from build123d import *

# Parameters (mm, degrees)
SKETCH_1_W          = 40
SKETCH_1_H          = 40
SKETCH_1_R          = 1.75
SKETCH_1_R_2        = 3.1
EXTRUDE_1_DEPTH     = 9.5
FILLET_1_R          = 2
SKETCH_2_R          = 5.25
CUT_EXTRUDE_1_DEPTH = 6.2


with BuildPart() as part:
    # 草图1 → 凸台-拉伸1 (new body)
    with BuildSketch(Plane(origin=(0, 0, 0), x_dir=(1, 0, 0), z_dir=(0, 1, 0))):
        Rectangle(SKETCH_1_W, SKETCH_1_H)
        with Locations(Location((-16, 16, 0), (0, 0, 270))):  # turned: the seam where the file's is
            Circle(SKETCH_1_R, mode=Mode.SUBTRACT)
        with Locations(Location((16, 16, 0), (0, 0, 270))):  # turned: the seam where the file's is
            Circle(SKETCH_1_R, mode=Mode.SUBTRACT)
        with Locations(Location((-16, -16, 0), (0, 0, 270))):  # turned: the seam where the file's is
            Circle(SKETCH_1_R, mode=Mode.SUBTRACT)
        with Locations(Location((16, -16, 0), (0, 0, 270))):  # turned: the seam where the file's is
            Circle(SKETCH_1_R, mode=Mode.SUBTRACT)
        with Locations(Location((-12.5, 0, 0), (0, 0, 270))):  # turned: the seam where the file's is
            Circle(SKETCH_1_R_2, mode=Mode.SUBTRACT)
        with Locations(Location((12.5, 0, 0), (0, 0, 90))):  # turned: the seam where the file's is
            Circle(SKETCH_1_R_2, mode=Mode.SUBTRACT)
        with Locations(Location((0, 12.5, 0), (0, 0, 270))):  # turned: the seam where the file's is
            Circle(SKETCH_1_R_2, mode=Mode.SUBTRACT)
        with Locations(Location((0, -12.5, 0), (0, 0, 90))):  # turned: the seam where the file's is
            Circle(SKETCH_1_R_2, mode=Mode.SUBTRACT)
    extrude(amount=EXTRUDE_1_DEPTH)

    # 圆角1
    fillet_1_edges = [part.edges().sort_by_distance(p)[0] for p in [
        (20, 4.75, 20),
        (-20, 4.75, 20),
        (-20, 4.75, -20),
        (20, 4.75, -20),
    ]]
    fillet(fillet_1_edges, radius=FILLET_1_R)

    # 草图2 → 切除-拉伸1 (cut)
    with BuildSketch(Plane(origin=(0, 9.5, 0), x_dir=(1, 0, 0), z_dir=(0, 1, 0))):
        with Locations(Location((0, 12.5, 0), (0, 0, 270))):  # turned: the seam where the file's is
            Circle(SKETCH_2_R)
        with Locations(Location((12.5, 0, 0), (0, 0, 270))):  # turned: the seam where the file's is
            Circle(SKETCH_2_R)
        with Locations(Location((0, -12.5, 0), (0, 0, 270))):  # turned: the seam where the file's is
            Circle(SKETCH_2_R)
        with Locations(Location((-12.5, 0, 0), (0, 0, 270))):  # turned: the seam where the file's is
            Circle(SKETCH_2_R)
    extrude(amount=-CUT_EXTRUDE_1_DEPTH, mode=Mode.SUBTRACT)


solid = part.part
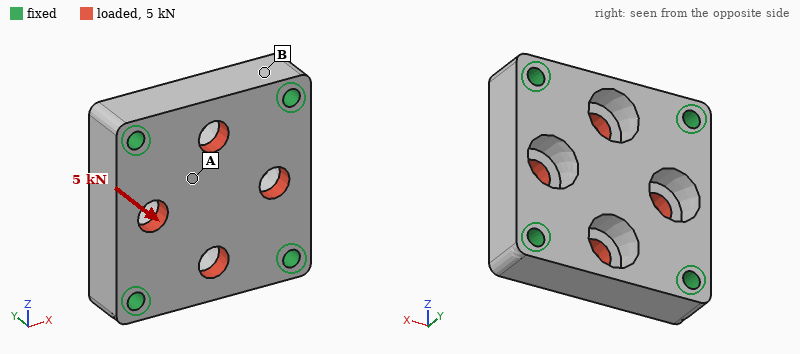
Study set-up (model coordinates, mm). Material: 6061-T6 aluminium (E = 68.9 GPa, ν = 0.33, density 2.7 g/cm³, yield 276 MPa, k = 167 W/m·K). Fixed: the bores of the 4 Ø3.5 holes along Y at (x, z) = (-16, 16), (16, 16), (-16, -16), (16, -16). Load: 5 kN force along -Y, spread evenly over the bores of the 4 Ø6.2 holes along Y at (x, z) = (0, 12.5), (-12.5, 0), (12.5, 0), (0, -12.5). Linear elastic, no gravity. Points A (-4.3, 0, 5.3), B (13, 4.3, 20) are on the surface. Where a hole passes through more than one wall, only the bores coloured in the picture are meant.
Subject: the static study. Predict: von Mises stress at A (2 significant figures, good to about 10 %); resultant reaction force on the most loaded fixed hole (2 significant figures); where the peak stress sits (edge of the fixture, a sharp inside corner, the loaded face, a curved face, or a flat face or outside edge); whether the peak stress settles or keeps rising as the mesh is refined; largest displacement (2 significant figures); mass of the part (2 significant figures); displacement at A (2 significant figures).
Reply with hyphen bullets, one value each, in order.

- 23 MPa
- 1.3 kN
- edge of the fixture
- keeps rising
- 16 µm
- 33 g
- 12 µm
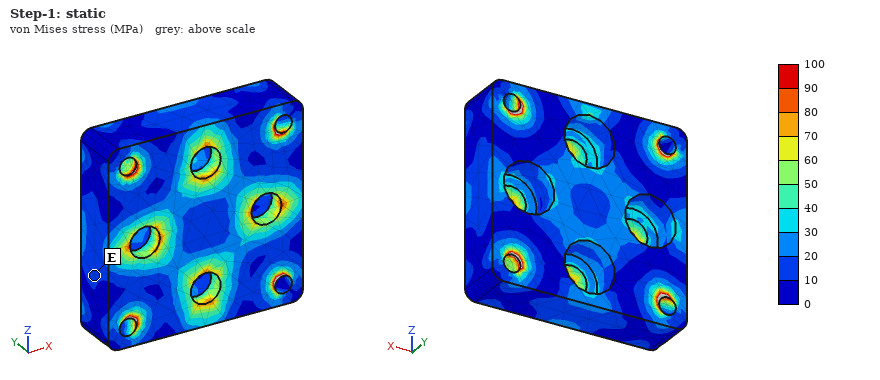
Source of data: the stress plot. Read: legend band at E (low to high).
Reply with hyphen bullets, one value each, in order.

- 10 to 20 MPa
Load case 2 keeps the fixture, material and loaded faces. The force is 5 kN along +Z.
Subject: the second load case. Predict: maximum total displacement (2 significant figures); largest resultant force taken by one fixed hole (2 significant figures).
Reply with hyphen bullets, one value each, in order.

- 8.0 µm
- 1.3 kN
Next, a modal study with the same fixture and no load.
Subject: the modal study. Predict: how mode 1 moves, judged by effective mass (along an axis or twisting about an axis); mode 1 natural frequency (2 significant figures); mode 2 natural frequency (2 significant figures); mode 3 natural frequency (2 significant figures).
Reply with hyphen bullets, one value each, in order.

- along Y
- 24 kHz
- 38 kHz
- 38 kHz
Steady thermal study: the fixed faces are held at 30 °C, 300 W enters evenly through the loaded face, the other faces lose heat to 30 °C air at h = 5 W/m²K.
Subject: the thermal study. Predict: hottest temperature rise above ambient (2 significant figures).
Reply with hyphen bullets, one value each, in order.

- 55 K
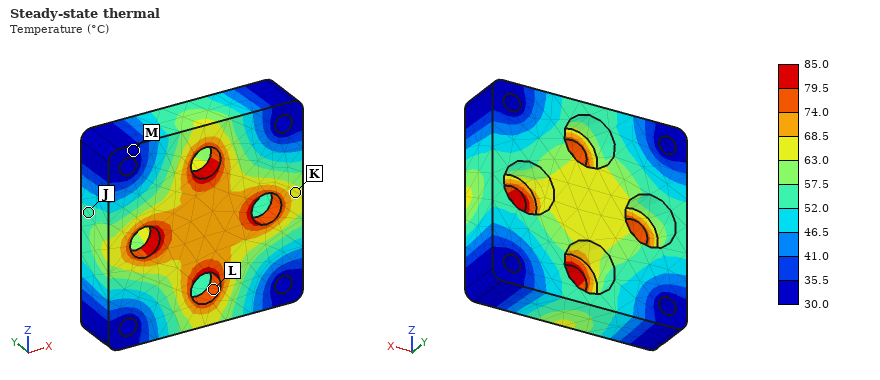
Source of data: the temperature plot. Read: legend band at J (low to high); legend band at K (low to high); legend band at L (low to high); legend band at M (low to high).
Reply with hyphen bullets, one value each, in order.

- 52.0 to 57.5 °C
- 63.0 to 68.5 °C
- 74.0 to 79.5 °C
- 30.0 to 35.5 °C
